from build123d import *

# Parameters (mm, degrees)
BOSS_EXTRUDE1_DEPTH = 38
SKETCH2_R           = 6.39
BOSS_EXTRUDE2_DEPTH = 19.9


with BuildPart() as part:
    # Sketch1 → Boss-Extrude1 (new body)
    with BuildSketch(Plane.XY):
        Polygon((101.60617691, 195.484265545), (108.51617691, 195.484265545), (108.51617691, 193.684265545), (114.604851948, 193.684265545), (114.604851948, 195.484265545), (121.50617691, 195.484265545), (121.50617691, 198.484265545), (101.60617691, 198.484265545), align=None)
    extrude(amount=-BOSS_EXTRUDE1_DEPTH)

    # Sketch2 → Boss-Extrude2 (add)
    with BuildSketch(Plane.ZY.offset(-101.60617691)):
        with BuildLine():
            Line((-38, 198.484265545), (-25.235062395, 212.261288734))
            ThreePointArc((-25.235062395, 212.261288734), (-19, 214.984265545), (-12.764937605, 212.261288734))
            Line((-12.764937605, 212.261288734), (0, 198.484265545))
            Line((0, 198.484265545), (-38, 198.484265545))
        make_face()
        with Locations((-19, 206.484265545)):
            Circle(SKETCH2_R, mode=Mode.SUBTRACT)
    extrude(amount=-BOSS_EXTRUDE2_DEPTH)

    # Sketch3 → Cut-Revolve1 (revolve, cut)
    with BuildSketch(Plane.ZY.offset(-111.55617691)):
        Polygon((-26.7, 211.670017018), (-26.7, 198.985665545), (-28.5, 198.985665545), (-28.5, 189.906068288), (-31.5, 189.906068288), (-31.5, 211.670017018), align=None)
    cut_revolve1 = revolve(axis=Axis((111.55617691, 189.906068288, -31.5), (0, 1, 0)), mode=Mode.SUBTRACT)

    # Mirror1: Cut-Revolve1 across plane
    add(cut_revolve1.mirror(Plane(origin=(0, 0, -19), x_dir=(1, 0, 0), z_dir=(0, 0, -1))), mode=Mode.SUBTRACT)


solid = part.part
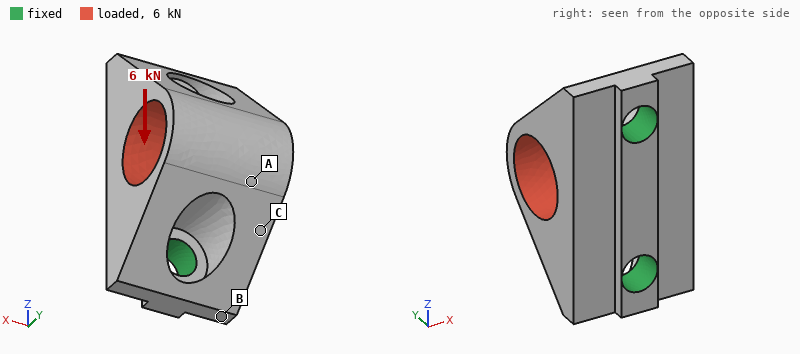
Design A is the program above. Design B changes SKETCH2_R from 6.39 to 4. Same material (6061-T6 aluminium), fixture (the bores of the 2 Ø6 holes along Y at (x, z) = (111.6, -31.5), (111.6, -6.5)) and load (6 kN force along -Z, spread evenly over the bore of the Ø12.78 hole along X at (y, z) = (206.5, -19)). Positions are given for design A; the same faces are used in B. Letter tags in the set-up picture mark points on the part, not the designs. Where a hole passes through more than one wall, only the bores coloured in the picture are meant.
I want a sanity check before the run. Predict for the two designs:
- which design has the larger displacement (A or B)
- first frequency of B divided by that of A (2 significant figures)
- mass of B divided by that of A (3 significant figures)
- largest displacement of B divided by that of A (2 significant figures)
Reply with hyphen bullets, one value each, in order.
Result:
- A
- 0.85
- 1.25
- 0.44
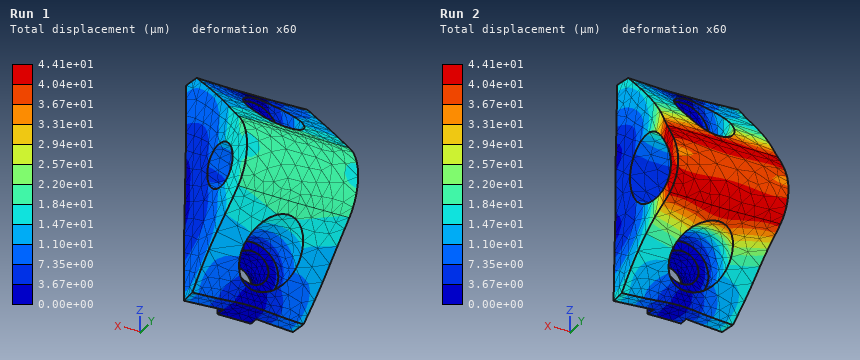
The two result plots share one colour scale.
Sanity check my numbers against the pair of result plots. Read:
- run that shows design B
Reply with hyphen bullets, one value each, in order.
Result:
- Run 1
